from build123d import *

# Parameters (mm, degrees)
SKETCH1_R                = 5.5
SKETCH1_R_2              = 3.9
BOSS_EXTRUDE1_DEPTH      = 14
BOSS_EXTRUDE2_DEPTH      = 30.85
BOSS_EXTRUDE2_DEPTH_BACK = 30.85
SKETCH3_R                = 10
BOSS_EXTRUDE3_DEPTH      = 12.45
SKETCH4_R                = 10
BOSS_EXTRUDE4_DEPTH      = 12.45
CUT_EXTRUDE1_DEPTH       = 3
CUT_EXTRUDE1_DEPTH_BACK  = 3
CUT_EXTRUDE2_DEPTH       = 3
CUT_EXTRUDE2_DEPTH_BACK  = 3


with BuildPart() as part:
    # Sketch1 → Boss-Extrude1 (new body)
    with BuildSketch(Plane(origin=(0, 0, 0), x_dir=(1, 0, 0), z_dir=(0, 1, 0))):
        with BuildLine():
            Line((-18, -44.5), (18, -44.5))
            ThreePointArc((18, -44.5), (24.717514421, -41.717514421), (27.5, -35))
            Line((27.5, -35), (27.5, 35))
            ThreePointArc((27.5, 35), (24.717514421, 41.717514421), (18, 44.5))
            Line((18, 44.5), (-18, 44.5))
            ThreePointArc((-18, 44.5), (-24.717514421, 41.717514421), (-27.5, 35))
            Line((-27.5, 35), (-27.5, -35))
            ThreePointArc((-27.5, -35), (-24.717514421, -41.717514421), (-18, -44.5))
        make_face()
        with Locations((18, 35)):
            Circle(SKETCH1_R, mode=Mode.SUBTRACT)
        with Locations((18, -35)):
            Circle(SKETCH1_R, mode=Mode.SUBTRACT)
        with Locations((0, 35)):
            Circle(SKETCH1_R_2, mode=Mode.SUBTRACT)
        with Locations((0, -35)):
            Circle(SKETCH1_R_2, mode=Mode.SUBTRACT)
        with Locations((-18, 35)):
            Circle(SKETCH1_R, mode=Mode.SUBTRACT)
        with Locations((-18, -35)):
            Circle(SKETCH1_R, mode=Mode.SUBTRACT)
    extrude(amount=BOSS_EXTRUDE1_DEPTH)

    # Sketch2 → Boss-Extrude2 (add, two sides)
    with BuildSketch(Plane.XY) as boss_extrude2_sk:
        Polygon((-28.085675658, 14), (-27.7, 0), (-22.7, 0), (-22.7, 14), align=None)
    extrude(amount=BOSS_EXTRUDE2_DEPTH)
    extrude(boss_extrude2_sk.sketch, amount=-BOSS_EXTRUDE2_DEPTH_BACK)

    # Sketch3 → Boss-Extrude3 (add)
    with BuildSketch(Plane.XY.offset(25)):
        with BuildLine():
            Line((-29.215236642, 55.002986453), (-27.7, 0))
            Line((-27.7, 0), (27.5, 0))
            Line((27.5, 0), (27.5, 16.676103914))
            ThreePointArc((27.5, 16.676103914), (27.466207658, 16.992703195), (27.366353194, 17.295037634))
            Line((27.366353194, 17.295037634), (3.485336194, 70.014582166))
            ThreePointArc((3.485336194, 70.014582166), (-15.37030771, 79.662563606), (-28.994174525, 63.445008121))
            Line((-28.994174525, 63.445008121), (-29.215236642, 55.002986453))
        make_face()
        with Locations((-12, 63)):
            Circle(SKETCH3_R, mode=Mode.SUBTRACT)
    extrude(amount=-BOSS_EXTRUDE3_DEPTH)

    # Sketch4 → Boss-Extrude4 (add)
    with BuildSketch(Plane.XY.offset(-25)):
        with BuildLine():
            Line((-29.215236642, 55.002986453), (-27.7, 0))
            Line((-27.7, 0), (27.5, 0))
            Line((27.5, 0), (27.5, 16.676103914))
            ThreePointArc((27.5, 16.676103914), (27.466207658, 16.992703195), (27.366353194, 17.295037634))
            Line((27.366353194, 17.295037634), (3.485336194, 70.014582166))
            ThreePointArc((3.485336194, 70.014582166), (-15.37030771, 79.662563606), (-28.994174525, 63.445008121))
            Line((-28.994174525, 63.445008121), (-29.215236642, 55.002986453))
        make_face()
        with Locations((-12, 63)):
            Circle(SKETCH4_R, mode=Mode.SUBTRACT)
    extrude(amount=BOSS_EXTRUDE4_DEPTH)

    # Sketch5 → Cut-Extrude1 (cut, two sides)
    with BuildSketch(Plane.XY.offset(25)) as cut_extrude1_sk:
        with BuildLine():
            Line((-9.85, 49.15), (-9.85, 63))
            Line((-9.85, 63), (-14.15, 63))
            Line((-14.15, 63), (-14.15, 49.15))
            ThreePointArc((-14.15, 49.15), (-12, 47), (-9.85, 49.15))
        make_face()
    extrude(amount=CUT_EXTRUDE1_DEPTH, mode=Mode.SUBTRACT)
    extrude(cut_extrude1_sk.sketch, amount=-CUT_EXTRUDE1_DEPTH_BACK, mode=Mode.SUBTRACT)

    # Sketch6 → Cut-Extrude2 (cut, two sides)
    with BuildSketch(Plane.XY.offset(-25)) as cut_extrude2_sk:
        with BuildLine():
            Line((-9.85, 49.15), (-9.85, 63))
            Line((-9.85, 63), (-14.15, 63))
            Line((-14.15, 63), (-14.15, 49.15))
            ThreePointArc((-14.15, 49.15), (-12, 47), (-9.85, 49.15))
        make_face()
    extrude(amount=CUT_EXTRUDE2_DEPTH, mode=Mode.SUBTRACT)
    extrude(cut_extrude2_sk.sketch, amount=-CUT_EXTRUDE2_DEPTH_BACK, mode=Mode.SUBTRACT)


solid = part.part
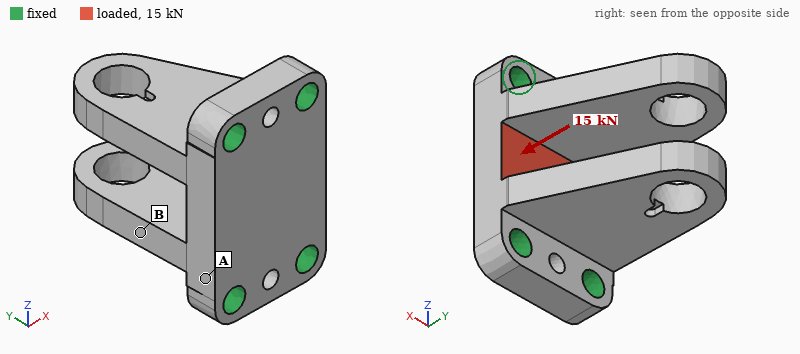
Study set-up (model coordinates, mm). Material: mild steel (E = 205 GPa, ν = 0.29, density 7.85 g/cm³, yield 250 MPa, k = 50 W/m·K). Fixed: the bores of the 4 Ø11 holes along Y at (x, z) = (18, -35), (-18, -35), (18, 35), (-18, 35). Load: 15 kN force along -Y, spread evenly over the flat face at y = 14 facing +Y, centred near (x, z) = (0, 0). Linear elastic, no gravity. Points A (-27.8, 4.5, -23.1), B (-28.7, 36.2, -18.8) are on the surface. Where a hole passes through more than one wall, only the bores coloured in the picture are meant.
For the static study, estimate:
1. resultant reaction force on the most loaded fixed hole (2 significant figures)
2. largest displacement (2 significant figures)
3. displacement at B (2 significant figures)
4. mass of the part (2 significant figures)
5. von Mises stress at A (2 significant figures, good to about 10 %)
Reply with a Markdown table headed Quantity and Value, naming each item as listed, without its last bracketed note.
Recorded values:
| Quantity | Value |
|---|---|
| resultant reaction force on the most loaded fixed hole | 3.8 kN |
| largest displacement | 32 µm |
| displacement at B | 13 µm |
| mass of the part | 950 g |
| von Mises stress at A | 27 MPa |
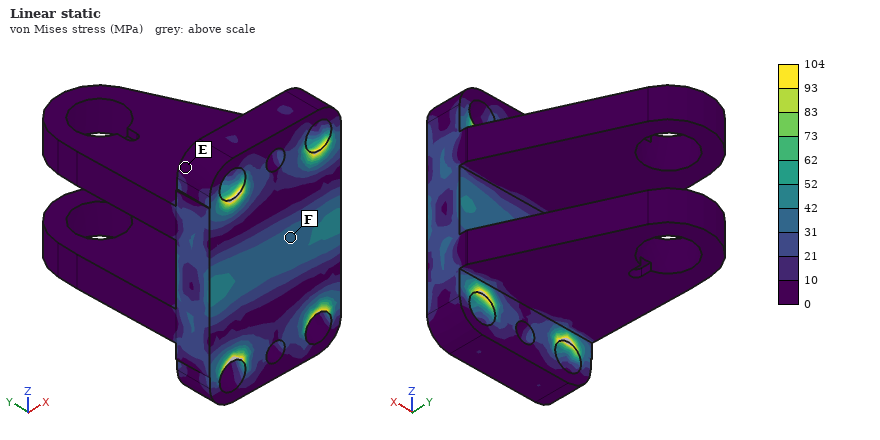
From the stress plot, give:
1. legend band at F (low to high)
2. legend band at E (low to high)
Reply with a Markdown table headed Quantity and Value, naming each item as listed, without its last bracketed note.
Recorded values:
| Quantity | Value |
|---|---|
| legend band at F | 31 to 42 MPa |
| legend band at E | 0 to 10 MPa |
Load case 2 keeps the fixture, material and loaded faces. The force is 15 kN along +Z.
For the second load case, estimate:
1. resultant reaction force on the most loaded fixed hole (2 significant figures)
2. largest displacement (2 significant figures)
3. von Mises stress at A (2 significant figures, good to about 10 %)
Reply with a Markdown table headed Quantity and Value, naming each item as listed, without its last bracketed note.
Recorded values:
| Quantity | Value |
|---|---|
| resultant reaction force on the most loaded fixed hole | 4.0 kN |
| largest displacement | 2.2 µm |
| von Mises stress at A | 7.4 MPa |
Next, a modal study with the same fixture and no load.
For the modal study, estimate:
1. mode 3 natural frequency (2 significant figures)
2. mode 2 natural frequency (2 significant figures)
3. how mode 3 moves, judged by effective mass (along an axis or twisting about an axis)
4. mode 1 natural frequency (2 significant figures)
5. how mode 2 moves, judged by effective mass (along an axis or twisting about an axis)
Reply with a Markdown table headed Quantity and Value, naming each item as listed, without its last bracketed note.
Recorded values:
| Quantity | Value |
|---|---|
| mode 3 natural frequency | 6000 Hz |
| mode 2 natural frequency | 3000 Hz |
| how mode 3 moves, judged by effective mass | along X |
| mode 1 natural frequency | 2700 Hz |
| how mode 2 moves, judged by effective mass | along Z |
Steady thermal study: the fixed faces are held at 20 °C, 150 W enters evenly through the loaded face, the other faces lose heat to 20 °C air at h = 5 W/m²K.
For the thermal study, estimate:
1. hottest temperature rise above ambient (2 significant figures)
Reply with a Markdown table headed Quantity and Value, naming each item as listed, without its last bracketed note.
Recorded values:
| Quantity | Value |
|---|---|
| hottest temperature rise above ambient | 57 K |
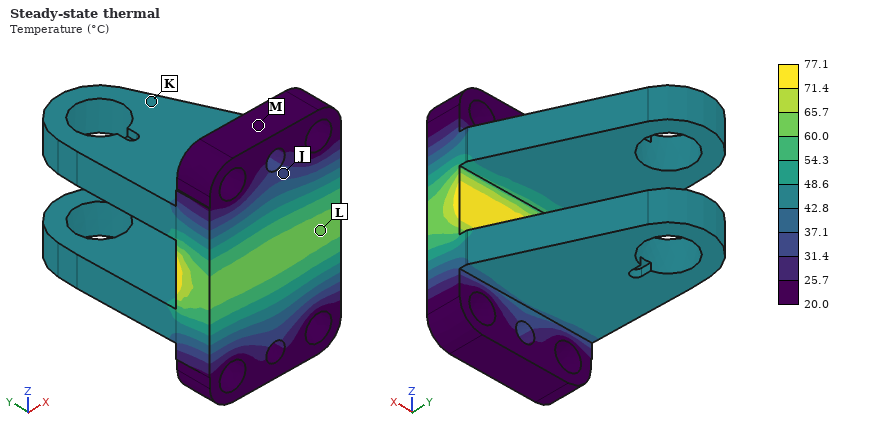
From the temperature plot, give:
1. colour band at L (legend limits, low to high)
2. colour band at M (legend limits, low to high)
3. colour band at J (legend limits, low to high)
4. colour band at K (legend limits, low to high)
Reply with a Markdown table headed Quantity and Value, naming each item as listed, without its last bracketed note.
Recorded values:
| Quantity | Value |
|---|---|
| colour band at L | 60.0 to 65.7 °C |
| colour band at M | 20.0 to 25.7 °C |
| colour band at J | 31.4 to 37.1 °C |
| colour band at K | 42.8 to 48.6 °C |
